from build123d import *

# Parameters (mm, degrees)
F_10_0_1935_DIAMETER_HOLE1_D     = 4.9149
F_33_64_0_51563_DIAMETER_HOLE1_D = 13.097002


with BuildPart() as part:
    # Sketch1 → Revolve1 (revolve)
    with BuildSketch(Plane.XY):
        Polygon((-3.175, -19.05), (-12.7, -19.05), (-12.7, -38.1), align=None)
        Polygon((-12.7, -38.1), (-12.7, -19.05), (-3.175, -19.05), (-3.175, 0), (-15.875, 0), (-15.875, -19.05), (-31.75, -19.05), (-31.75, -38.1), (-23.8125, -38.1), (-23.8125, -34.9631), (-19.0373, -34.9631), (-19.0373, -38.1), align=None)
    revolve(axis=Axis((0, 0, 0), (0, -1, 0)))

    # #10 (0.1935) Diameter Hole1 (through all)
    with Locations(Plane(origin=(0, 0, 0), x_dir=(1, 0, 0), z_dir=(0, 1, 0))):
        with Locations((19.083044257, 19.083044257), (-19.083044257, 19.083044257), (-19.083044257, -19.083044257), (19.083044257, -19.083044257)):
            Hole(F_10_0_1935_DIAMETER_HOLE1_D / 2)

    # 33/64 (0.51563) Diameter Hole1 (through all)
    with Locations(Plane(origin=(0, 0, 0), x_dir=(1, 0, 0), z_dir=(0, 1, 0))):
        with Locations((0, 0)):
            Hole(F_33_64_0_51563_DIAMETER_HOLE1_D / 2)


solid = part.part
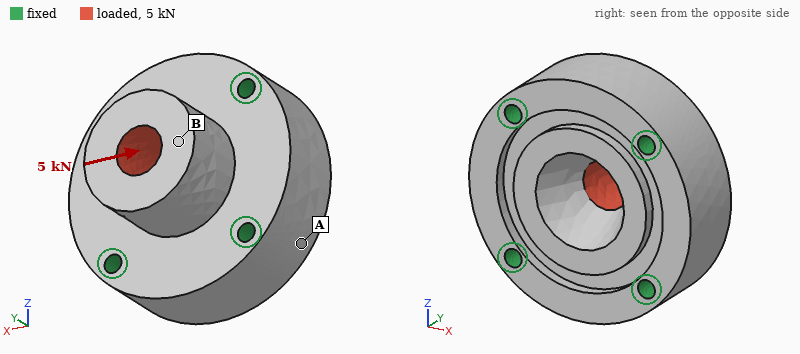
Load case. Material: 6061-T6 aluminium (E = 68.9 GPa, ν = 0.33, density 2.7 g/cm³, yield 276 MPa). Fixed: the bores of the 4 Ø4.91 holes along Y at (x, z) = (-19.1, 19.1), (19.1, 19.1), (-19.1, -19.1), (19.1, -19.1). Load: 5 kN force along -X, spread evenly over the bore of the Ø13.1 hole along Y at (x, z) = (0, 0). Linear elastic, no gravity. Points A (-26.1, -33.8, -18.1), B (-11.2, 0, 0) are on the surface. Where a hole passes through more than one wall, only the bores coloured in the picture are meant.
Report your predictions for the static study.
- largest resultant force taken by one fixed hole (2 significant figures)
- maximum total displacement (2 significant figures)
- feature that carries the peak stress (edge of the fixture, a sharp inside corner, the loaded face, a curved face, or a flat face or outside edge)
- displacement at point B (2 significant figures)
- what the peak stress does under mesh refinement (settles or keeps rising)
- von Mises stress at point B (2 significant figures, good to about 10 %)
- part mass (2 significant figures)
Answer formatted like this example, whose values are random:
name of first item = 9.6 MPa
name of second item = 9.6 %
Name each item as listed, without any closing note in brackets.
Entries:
largest resultant force taken by one fixed hole = 1.6 kN
maximum total displacement = 9.8 µm
feature that carries the peak stress = edge of the fixture
displacement at point B = 9.6 µm
what the peak stress does under mesh refinement = keeps rising
von Mises stress at point B = 7.1 MPa
part mass = 170 g
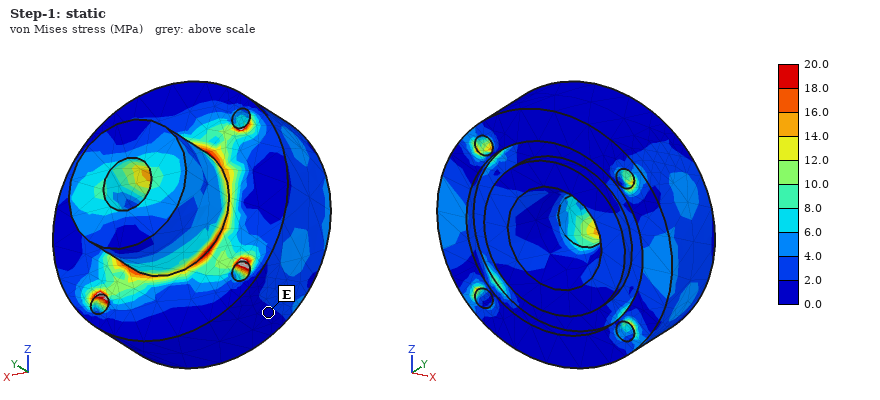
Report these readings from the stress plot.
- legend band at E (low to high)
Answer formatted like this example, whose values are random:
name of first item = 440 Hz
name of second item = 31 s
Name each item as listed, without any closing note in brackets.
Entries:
legend band at E = 0.0 to 2.0 MPa
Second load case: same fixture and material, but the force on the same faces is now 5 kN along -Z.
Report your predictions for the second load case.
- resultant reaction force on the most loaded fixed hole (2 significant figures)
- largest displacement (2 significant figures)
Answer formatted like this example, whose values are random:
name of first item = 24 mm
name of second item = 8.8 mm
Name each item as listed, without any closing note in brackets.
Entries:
resultant reaction force on the most loaded fixed hole = 1.6 kN
largest displacement = 9.8 µm
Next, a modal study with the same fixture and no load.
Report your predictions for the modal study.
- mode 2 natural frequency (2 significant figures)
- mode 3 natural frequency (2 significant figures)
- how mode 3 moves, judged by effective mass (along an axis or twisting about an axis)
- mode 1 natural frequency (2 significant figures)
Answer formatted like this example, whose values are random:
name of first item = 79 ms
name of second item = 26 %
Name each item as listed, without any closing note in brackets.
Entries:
mode 2 natural frequency = 19 kHz
mode 3 natural frequency = 22 kHz
how mode 3 moves, judged by effective mass = along Y
mode 1 natural frequency = 19 kHz
